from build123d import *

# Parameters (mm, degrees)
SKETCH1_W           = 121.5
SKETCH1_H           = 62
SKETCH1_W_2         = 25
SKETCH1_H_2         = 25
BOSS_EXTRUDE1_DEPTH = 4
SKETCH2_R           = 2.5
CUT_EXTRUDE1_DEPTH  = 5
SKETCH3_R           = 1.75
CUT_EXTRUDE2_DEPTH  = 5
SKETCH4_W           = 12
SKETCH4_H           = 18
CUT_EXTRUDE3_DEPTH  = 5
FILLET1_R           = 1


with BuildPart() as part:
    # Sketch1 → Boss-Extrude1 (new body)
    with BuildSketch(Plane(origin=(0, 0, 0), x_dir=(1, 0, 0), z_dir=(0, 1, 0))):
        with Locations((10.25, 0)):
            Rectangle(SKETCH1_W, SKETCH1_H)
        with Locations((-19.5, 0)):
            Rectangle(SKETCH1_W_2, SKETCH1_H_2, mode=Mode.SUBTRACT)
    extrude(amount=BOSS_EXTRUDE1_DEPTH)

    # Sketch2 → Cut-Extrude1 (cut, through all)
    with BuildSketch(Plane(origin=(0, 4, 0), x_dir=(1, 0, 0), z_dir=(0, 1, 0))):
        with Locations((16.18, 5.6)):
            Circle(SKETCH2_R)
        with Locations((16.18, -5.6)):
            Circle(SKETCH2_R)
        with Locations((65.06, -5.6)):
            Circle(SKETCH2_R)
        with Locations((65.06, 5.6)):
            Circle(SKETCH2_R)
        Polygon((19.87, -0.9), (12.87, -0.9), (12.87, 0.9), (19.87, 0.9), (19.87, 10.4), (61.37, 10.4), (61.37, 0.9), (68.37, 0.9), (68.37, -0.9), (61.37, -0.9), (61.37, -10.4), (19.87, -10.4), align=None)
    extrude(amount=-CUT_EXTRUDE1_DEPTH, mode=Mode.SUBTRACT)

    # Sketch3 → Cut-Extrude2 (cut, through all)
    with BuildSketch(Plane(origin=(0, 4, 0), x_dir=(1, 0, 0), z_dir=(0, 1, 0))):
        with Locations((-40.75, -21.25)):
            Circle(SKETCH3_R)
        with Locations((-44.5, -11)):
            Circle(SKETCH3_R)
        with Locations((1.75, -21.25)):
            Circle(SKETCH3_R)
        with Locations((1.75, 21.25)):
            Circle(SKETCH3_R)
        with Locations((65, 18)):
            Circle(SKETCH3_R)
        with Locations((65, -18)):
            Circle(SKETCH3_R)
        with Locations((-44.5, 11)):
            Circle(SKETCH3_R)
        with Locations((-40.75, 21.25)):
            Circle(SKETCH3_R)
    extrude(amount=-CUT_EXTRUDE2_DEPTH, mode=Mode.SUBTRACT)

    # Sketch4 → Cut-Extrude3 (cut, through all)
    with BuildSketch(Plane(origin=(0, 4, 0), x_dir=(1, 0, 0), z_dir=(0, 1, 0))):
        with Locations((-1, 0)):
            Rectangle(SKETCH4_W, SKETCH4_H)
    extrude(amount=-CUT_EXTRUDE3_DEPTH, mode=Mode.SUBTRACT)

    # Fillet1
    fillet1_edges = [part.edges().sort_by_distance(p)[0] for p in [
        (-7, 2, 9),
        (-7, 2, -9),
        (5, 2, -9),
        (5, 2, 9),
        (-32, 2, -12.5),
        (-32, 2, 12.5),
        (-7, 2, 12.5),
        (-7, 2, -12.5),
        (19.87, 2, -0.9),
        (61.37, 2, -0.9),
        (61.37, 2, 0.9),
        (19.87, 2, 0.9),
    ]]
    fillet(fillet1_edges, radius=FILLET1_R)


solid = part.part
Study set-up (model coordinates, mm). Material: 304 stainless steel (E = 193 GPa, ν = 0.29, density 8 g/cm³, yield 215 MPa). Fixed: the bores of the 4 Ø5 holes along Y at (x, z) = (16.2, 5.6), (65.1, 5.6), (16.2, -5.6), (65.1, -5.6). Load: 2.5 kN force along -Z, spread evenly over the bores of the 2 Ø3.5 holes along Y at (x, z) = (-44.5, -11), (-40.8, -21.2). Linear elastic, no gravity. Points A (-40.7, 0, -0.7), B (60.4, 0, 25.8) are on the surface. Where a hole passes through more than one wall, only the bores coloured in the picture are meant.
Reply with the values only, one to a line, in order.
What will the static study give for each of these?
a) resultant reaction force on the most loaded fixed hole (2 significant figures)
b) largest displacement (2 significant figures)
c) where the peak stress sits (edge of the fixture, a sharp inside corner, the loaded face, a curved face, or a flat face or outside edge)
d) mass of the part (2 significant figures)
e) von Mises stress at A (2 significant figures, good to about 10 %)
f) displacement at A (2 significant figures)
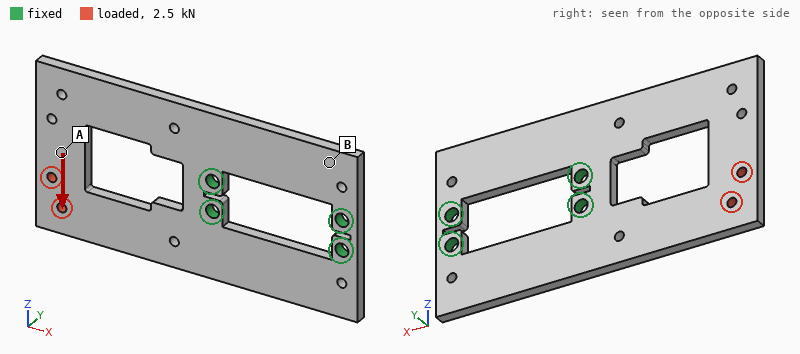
2.4 kN
0.10 mm
a curved face
180 g
51 MPa
0.087 mm
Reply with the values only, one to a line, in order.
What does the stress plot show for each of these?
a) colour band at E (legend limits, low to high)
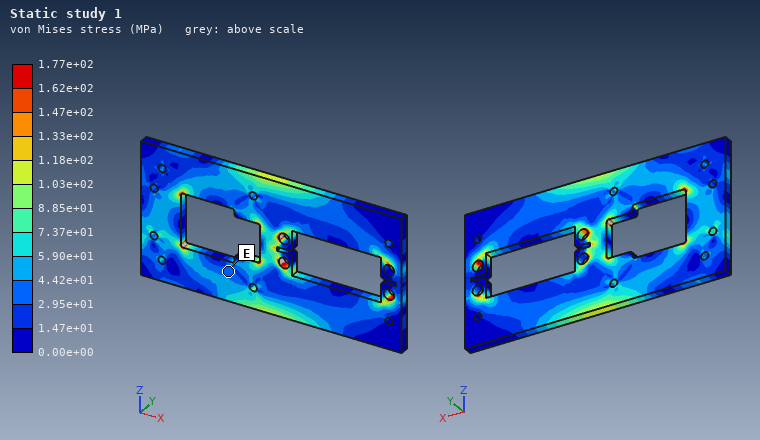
2.95e+01 to 4.42e+01 MPa
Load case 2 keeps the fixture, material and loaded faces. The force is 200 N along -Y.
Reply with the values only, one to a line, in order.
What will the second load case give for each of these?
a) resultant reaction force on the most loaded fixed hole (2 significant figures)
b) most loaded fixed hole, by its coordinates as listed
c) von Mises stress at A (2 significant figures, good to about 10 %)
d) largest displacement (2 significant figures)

240 N
(16.2, -5.6)
20 MPa
0.50 mm
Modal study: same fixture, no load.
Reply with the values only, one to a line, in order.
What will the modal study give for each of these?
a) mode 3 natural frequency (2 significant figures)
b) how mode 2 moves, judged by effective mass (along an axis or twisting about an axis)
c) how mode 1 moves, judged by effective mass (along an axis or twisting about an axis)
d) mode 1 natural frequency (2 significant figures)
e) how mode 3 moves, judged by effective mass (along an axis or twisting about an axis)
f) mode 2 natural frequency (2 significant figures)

3000 Hz
twisting about X
along Y
600 Hz
along Y
1300 Hz
